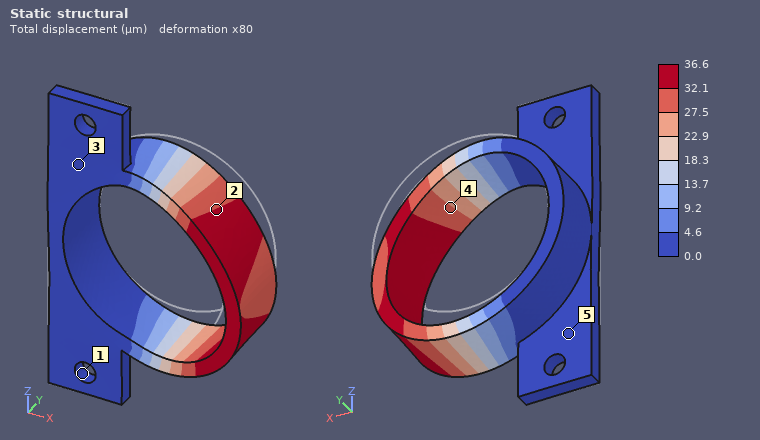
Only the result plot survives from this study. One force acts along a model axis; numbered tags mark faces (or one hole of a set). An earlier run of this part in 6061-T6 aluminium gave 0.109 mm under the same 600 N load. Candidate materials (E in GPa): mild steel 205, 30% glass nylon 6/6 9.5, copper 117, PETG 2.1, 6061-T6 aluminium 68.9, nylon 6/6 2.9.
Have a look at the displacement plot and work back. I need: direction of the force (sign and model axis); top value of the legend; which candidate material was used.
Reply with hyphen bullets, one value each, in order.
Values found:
- -Z
- 36.6 µm
- mild steel
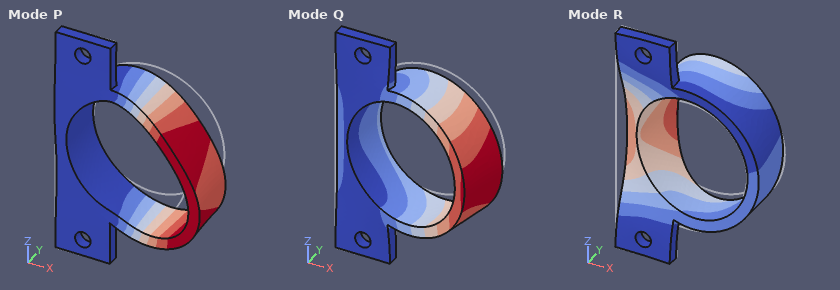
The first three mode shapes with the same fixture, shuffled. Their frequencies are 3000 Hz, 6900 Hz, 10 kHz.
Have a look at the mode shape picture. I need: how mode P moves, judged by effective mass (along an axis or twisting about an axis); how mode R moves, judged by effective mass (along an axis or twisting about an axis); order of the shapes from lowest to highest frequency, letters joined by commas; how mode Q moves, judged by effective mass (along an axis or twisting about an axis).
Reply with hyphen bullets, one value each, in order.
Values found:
- along Z
- along Y
- Q, P, R
- along Y
